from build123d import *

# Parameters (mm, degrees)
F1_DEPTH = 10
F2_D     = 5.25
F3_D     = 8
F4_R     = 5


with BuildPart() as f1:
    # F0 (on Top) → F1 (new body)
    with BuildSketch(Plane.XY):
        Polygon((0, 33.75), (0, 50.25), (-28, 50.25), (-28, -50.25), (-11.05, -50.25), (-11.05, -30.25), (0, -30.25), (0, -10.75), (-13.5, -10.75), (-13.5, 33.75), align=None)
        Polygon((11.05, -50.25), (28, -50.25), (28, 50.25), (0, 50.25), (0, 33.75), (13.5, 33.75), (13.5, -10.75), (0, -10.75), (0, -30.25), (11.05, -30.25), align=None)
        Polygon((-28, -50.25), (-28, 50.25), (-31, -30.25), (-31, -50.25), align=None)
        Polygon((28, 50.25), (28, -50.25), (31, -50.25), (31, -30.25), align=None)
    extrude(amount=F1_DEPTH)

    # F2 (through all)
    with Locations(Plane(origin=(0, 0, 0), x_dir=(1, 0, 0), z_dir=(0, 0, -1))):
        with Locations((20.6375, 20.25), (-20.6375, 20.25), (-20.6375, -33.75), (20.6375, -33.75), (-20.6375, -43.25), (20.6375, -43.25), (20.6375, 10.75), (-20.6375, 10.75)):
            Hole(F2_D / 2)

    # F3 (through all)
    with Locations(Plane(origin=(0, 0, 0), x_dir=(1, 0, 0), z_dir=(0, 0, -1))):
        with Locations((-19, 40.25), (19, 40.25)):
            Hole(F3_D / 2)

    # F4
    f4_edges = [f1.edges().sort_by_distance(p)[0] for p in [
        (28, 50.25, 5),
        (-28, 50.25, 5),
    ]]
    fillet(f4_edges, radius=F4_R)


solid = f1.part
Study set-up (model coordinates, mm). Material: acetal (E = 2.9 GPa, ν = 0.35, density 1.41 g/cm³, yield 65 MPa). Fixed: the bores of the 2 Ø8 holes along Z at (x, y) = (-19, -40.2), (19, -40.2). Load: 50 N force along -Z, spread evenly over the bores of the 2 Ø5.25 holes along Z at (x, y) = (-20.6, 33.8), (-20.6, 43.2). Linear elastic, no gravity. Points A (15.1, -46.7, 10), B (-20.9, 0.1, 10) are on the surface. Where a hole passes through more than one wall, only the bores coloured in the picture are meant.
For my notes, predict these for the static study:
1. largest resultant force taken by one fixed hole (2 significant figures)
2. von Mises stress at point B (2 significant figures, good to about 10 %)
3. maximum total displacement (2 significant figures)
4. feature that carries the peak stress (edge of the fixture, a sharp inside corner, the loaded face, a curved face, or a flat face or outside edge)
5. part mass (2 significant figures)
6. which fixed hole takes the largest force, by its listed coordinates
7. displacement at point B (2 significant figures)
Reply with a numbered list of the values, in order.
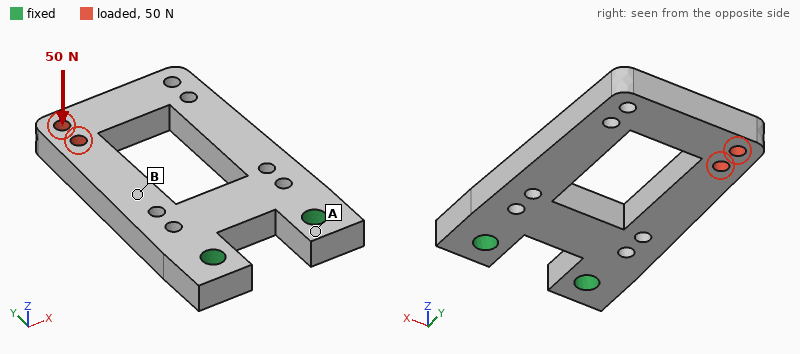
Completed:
1. 44 N
2. 4.0 MPa
3. 1.3 mm
4. a curved face
5. 57 g
6. (-19, -40.2)
7. 0.33 mm
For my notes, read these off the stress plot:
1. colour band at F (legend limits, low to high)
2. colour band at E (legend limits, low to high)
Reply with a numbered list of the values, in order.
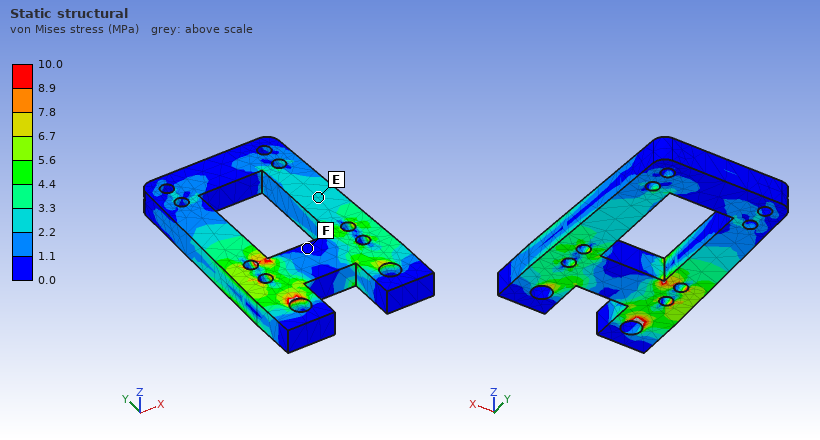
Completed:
1. 0.0 to 1.1 MPa
2. 2.2 to 3.3 MPa
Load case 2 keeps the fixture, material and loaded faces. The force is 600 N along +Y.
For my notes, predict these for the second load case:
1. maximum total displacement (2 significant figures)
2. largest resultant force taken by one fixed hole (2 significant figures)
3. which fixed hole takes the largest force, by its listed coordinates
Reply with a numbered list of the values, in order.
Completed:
1. 0.14 mm
2. 590 N
3. (-19, -40.2)
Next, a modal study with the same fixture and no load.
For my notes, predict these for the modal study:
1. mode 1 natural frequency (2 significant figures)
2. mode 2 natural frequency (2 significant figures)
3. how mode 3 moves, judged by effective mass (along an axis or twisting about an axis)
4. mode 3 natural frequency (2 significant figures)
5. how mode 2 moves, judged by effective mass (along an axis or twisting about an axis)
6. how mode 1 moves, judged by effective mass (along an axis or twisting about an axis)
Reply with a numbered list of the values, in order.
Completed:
1. 270 Hz
2. 740 Hz
3. along X
4. 870 Hz
5. twisting about Y
6. along Z
